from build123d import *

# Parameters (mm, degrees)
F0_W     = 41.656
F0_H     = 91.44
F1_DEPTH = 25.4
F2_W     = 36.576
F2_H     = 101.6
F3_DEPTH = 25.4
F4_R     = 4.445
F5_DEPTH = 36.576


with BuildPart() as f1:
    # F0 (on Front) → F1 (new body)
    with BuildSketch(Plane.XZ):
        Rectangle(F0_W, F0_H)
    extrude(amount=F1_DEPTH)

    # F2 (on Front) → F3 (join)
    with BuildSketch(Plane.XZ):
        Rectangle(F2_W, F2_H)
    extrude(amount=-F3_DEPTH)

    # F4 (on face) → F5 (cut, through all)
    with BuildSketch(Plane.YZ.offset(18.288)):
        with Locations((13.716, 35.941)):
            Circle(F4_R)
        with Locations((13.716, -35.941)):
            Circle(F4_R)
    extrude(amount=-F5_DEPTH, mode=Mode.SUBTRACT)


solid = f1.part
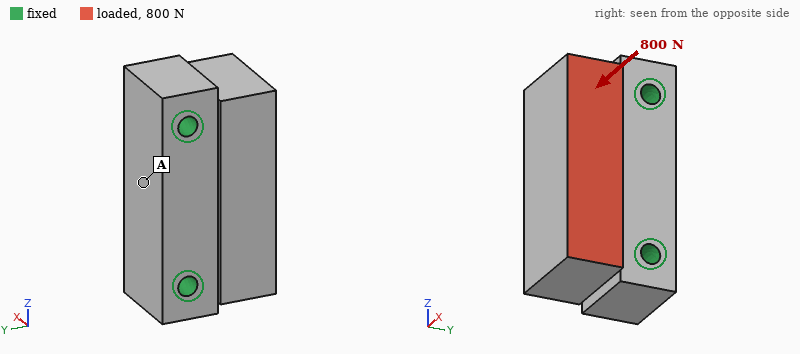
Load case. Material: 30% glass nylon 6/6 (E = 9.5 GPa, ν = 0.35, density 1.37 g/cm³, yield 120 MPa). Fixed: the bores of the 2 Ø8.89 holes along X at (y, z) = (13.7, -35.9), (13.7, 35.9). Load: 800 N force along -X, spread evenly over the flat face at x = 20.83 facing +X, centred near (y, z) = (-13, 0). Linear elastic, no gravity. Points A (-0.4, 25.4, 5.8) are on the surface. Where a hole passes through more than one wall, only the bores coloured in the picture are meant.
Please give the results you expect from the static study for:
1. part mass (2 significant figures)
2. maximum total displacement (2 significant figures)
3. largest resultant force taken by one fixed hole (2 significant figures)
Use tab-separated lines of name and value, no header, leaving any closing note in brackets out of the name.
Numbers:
part mass	260 g
maximum total displacement	9.6 µm
largest resultant force taken by one fixed hole	400 N
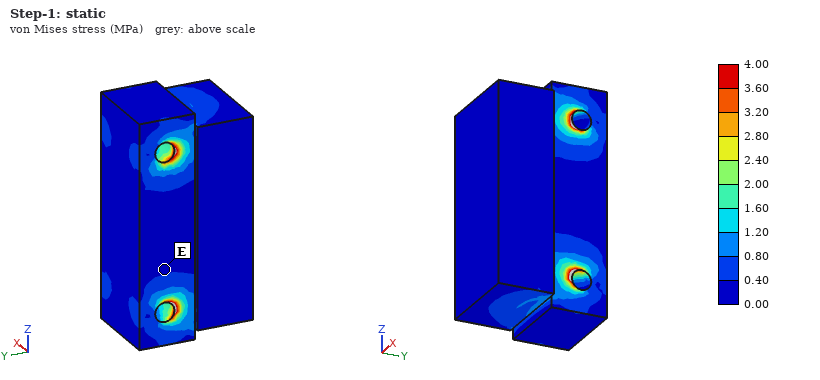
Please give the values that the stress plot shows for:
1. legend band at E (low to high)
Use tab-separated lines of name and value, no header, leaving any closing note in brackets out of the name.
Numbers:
legend band at E	0.00 to 0.40 MPa
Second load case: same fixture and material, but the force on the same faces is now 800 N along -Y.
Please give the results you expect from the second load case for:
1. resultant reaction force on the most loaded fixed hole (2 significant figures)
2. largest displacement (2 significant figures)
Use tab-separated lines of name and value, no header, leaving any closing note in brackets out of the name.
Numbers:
resultant reaction force on the most loaded fixed hole	420 N
largest displacement	9.2 µm
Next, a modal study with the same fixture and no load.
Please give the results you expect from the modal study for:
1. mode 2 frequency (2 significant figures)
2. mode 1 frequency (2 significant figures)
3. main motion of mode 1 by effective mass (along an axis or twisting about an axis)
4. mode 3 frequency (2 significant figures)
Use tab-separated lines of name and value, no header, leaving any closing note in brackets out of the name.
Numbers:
mode 2 frequency	7800 Hz
mode 1 frequency	4700 Hz
main motion of mode 1 by effective mass	along X
mode 3 frequency	8000 Hz
